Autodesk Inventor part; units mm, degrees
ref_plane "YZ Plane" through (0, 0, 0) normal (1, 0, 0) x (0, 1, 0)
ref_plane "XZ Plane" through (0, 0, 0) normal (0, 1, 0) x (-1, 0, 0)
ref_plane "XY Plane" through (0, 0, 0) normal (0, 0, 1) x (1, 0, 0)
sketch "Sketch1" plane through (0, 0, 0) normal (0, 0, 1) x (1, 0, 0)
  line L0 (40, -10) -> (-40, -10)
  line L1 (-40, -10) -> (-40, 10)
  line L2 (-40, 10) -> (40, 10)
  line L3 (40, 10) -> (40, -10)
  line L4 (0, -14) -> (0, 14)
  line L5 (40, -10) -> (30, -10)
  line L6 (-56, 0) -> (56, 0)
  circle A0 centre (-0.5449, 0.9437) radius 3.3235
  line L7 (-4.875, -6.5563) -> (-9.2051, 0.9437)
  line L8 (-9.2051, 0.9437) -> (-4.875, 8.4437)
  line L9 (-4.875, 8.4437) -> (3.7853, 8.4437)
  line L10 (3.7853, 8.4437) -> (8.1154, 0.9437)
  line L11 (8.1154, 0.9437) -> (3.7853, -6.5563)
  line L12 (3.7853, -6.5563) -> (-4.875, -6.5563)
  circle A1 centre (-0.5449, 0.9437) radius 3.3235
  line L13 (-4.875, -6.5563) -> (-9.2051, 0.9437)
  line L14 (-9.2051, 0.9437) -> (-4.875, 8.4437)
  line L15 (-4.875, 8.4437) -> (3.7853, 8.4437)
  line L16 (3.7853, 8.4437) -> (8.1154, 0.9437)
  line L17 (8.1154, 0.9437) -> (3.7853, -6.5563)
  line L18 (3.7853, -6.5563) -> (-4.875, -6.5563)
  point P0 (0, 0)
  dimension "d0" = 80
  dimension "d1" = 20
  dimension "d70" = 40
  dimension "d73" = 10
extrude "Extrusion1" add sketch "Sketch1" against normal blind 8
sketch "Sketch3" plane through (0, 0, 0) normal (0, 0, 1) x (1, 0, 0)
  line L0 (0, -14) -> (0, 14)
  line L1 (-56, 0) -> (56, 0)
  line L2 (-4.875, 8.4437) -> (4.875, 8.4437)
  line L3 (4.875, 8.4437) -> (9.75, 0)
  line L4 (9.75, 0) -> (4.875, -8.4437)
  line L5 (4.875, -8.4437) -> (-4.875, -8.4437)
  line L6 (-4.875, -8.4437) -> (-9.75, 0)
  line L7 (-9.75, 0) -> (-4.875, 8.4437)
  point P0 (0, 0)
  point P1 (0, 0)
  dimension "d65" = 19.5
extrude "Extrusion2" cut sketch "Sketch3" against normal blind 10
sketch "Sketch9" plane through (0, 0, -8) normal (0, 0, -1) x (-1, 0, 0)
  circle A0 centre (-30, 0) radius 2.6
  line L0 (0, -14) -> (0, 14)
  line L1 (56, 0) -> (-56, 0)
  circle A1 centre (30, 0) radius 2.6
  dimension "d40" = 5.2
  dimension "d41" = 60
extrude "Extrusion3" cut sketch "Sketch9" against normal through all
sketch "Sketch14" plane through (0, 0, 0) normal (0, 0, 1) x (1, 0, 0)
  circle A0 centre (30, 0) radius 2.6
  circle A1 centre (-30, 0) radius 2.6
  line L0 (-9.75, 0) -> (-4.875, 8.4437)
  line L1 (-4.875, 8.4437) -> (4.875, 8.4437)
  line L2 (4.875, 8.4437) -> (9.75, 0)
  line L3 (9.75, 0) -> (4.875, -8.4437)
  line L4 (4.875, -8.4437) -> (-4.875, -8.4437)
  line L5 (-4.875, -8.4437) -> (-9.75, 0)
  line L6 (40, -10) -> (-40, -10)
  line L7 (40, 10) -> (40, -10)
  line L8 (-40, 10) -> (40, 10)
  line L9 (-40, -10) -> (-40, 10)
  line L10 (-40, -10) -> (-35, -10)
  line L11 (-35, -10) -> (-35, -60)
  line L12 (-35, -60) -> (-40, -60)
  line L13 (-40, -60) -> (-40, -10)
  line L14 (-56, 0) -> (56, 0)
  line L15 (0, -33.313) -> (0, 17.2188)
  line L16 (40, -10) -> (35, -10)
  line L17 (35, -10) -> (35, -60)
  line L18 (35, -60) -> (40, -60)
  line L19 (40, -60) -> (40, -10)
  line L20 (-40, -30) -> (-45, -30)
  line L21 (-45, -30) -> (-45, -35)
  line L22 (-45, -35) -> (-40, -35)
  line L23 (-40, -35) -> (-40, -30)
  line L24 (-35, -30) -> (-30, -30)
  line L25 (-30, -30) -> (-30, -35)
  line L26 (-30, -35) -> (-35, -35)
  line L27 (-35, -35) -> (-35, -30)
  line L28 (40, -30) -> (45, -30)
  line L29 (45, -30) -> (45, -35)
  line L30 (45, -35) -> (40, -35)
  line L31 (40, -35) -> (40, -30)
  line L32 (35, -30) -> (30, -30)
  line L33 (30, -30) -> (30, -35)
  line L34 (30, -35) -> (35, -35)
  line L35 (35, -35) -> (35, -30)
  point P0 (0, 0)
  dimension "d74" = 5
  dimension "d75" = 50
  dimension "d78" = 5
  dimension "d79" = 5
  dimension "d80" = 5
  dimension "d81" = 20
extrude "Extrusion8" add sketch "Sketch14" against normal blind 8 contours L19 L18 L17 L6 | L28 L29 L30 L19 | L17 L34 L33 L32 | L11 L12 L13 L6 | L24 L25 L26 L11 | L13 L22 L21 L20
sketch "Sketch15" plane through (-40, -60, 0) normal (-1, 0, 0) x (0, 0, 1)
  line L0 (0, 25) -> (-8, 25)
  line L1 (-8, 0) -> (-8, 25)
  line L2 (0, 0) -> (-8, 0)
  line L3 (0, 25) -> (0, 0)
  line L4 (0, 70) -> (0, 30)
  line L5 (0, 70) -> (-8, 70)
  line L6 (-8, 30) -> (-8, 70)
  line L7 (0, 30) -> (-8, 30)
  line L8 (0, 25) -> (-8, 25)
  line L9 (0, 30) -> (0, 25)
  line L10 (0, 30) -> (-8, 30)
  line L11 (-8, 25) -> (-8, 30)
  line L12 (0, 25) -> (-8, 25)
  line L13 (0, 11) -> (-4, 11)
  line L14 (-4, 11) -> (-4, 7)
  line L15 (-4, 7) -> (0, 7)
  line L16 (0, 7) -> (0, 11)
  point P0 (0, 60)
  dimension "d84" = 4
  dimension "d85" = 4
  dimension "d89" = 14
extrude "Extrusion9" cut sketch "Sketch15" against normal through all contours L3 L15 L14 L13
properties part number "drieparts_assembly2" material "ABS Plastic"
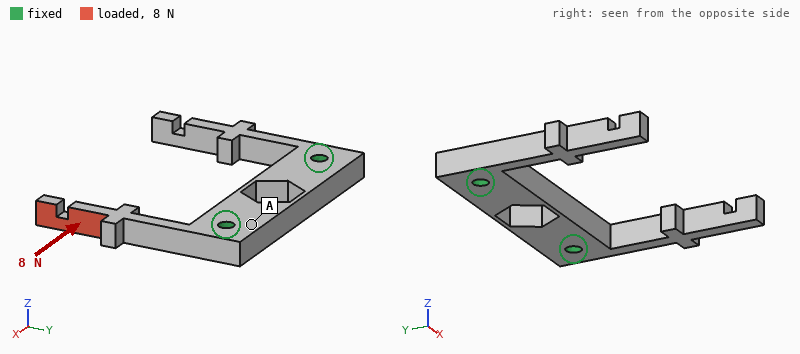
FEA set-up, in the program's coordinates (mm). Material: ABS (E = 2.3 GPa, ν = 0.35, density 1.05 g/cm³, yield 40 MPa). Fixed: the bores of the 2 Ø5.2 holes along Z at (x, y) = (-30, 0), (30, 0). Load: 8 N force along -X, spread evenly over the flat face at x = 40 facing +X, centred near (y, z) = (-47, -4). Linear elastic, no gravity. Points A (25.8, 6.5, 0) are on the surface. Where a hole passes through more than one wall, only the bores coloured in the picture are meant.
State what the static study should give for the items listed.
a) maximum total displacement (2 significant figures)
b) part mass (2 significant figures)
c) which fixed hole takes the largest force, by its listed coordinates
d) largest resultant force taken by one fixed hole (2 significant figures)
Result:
1.3 mm
16 g
(30, 0)
7.2 N
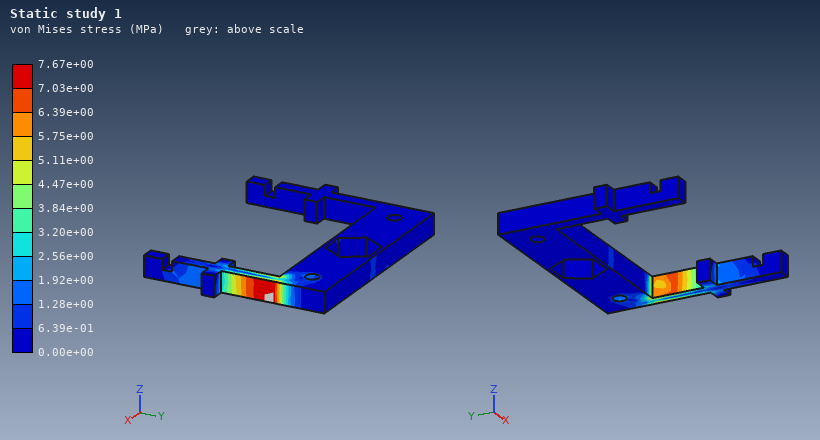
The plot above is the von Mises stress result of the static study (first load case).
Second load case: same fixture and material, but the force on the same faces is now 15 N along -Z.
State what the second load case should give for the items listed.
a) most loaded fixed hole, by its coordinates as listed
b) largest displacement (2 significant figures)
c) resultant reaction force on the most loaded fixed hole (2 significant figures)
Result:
(30, 0)
1.3 mm
16 N
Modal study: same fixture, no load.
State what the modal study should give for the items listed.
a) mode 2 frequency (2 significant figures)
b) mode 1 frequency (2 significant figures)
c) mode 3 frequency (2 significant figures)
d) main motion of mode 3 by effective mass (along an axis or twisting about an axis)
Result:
430 Hz
430 Hz
590 Hz
along Z
